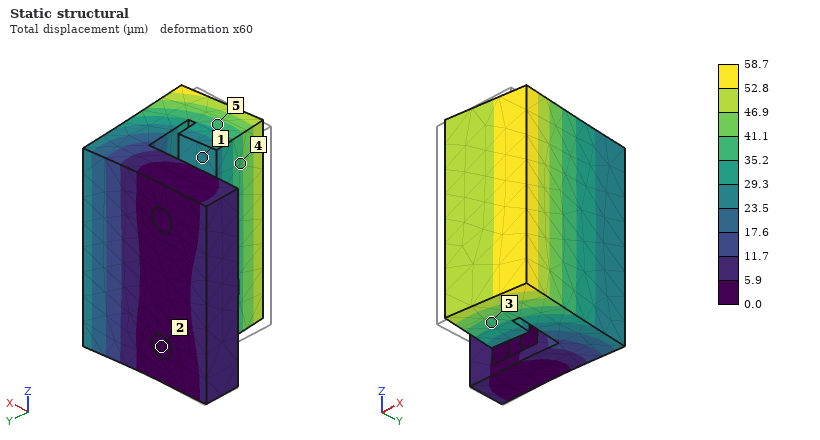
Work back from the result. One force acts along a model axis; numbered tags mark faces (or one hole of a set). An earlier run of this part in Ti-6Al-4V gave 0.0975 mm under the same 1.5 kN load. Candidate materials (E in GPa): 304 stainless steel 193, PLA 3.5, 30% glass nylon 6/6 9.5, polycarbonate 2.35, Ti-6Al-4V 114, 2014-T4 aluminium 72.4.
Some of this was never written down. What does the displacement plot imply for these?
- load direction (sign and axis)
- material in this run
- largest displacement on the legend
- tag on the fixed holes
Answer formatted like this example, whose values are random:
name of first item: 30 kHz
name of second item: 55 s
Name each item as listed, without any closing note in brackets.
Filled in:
load direction: +X
material in this run: 304 stainless steel
largest displacement on the legend: 58.7 µm
tag on the fixed holes: 2
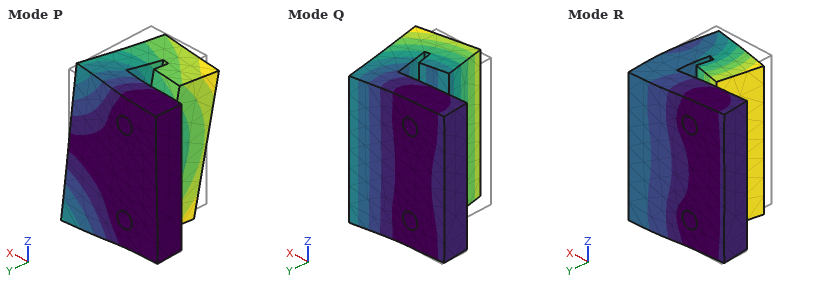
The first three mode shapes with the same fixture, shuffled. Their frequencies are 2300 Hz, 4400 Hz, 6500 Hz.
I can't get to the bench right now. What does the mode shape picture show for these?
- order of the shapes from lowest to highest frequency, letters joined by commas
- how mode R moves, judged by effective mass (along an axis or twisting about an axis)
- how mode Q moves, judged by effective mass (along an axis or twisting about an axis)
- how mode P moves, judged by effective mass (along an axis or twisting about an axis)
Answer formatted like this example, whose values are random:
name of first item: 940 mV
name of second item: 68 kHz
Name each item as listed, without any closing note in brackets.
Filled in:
order of the shapes from lowest to highest frequency, letters joined by commas: Q, P, R
how mode R moves, judged by effective mass: along Y
how mode Q moves, judged by effective mass: along X
how mode P moves, judged by effective mass: along Z
